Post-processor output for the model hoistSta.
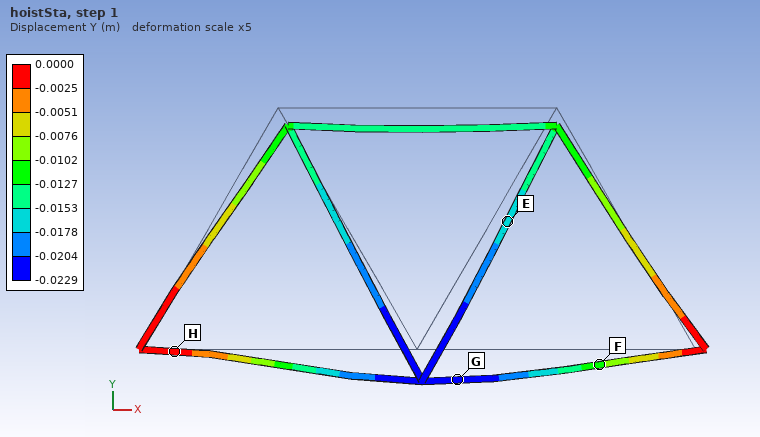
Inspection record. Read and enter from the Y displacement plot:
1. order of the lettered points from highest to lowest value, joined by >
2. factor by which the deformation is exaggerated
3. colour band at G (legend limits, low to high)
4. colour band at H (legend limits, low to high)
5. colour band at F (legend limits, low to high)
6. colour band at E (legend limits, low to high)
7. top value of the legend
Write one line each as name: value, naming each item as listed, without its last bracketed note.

order of the lettered points from highest to lowest value, joined by >: H > F > E > G
factor by which the deformation is exaggerated: 5
colour band at G: -0.0229 to -0.0204 m
colour band at H: -0.0025 to 0.0000 m
colour band at F: -0.0127 to -0.0102 m
colour band at E: -0.0178 to -0.0153 m
top value of the legend: 0.0000 m
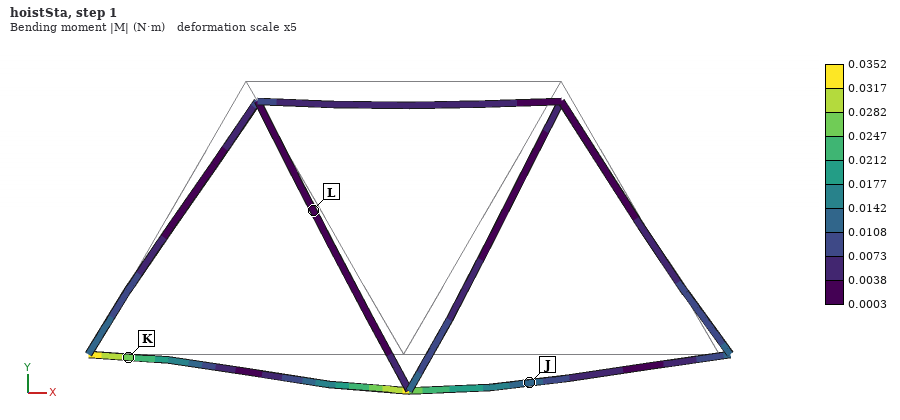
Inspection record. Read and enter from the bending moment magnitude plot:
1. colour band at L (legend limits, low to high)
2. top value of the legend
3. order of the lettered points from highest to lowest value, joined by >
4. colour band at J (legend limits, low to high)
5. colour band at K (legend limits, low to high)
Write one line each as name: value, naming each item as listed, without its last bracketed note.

colour band at L: 0.0003 to 0.0038 N·m
top value of the legend: 0.0352 N·m
order of the lettered points from highest to lowest value, joined by >: K > J > L
colour band at J: 0.0108 to 0.0142 N·m
colour band at K: 0.0247 to 0.0282 N·m
